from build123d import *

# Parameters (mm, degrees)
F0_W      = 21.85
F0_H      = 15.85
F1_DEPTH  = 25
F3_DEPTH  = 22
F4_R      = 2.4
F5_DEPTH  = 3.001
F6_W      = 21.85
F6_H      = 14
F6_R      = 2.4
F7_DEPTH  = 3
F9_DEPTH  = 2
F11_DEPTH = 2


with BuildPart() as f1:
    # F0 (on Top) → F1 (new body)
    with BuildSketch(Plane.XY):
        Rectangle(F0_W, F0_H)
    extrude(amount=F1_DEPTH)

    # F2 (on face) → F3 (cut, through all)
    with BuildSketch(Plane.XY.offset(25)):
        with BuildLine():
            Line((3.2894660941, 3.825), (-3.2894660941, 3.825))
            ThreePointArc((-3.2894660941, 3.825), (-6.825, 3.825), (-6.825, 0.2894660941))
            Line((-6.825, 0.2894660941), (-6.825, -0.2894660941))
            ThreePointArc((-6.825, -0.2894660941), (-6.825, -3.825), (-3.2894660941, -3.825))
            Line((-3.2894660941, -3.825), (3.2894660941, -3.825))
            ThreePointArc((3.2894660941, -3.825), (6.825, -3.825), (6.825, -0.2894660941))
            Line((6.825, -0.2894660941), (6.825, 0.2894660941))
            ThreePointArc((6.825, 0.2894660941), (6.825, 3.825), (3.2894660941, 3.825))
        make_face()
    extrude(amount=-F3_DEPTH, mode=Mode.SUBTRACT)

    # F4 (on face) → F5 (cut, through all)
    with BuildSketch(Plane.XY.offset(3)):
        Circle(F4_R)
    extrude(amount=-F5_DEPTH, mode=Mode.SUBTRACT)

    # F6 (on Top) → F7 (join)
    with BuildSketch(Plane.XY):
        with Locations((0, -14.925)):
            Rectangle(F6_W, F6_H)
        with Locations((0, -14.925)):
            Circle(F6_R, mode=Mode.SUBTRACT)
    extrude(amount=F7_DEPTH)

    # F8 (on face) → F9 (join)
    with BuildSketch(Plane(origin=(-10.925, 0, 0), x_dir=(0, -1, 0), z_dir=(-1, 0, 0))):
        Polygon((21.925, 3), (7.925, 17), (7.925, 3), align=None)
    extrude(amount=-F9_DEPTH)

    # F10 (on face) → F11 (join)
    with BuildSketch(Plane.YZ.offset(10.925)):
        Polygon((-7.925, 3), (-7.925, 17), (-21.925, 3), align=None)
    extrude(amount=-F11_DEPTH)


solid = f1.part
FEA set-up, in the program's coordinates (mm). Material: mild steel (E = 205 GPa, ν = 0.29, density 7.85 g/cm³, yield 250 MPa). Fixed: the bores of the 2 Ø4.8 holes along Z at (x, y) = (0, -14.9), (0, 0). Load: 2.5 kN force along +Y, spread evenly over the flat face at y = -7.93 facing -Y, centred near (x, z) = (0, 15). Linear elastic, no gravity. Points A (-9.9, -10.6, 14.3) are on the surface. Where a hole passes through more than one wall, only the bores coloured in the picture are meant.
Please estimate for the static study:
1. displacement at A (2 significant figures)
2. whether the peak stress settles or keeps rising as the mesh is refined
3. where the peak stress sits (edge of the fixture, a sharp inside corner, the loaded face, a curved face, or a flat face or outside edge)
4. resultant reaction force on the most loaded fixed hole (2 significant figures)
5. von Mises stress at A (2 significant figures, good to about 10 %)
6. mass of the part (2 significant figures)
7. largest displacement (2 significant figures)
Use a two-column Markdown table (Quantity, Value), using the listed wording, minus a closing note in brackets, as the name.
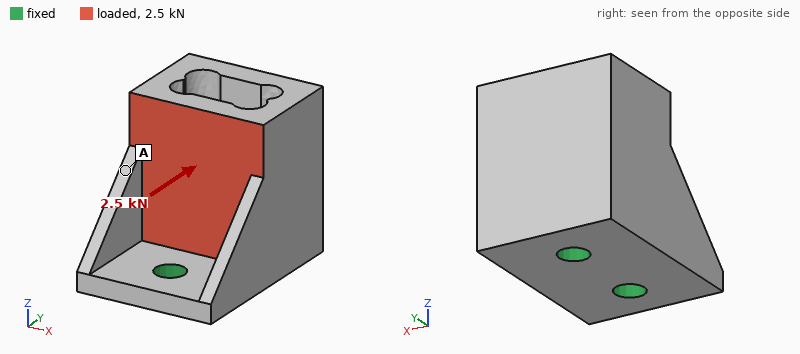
| Quantity | Value |
|---|---|
| displacement at A | 17 µm |
| whether the peak stress settles or keeps rising as the mesh is refined | keeps rising |
| where the peak stress sits | edge of the fixture |
| resultant reaction force on the most loaded fixed hole | 2.2 kN |
| von Mises stress at A | 43 MPa |
| mass of the part | 57 g |
| largest displacement | 32 µm |
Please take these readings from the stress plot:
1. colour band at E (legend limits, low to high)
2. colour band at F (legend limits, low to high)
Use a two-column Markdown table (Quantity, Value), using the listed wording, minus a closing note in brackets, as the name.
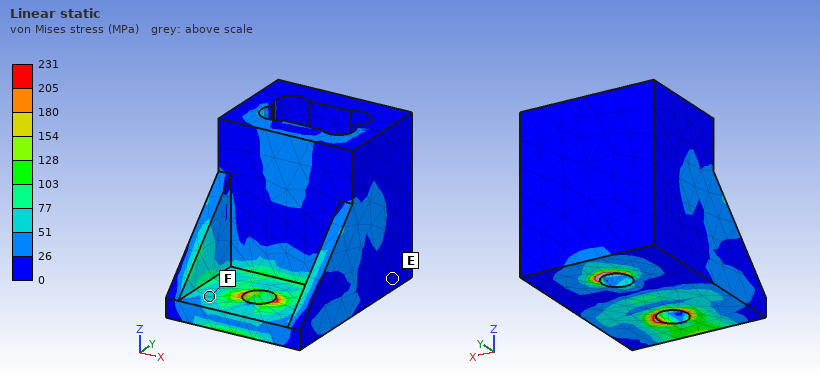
| Quantity | Value |
|---|---|
| colour band at E | 0 to 26 MPa |
| colour band at F | 51 to 77 MPa |
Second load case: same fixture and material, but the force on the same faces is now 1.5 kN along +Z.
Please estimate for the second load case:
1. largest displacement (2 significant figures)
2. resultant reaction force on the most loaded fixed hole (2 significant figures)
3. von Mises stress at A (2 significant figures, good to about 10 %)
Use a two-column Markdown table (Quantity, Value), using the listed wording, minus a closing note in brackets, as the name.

| Quantity | Value |
|---|---|
| largest displacement | 8.3 µm |
| resultant reaction force on the most loaded fixed hole | 800 N |
| von Mises stress at A | 18 MPa |
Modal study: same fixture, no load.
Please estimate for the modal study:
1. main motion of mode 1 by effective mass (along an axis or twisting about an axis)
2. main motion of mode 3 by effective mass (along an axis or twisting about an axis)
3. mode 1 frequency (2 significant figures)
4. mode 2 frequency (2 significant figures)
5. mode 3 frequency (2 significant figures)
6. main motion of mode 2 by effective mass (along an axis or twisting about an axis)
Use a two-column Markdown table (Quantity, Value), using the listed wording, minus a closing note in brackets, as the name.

| Quantity | Value |
|---|---|
| main motion of mode 1 by effective mass | along X |
| main motion of mode 3 by effective mass | twisting about Z |
| mode 1 frequency | 5500 Hz |
| mode 2 frequency | 8400 Hz |
| mode 3 frequency | 19 kHz |
| main motion of mode 2 by effective mass | along Y |
